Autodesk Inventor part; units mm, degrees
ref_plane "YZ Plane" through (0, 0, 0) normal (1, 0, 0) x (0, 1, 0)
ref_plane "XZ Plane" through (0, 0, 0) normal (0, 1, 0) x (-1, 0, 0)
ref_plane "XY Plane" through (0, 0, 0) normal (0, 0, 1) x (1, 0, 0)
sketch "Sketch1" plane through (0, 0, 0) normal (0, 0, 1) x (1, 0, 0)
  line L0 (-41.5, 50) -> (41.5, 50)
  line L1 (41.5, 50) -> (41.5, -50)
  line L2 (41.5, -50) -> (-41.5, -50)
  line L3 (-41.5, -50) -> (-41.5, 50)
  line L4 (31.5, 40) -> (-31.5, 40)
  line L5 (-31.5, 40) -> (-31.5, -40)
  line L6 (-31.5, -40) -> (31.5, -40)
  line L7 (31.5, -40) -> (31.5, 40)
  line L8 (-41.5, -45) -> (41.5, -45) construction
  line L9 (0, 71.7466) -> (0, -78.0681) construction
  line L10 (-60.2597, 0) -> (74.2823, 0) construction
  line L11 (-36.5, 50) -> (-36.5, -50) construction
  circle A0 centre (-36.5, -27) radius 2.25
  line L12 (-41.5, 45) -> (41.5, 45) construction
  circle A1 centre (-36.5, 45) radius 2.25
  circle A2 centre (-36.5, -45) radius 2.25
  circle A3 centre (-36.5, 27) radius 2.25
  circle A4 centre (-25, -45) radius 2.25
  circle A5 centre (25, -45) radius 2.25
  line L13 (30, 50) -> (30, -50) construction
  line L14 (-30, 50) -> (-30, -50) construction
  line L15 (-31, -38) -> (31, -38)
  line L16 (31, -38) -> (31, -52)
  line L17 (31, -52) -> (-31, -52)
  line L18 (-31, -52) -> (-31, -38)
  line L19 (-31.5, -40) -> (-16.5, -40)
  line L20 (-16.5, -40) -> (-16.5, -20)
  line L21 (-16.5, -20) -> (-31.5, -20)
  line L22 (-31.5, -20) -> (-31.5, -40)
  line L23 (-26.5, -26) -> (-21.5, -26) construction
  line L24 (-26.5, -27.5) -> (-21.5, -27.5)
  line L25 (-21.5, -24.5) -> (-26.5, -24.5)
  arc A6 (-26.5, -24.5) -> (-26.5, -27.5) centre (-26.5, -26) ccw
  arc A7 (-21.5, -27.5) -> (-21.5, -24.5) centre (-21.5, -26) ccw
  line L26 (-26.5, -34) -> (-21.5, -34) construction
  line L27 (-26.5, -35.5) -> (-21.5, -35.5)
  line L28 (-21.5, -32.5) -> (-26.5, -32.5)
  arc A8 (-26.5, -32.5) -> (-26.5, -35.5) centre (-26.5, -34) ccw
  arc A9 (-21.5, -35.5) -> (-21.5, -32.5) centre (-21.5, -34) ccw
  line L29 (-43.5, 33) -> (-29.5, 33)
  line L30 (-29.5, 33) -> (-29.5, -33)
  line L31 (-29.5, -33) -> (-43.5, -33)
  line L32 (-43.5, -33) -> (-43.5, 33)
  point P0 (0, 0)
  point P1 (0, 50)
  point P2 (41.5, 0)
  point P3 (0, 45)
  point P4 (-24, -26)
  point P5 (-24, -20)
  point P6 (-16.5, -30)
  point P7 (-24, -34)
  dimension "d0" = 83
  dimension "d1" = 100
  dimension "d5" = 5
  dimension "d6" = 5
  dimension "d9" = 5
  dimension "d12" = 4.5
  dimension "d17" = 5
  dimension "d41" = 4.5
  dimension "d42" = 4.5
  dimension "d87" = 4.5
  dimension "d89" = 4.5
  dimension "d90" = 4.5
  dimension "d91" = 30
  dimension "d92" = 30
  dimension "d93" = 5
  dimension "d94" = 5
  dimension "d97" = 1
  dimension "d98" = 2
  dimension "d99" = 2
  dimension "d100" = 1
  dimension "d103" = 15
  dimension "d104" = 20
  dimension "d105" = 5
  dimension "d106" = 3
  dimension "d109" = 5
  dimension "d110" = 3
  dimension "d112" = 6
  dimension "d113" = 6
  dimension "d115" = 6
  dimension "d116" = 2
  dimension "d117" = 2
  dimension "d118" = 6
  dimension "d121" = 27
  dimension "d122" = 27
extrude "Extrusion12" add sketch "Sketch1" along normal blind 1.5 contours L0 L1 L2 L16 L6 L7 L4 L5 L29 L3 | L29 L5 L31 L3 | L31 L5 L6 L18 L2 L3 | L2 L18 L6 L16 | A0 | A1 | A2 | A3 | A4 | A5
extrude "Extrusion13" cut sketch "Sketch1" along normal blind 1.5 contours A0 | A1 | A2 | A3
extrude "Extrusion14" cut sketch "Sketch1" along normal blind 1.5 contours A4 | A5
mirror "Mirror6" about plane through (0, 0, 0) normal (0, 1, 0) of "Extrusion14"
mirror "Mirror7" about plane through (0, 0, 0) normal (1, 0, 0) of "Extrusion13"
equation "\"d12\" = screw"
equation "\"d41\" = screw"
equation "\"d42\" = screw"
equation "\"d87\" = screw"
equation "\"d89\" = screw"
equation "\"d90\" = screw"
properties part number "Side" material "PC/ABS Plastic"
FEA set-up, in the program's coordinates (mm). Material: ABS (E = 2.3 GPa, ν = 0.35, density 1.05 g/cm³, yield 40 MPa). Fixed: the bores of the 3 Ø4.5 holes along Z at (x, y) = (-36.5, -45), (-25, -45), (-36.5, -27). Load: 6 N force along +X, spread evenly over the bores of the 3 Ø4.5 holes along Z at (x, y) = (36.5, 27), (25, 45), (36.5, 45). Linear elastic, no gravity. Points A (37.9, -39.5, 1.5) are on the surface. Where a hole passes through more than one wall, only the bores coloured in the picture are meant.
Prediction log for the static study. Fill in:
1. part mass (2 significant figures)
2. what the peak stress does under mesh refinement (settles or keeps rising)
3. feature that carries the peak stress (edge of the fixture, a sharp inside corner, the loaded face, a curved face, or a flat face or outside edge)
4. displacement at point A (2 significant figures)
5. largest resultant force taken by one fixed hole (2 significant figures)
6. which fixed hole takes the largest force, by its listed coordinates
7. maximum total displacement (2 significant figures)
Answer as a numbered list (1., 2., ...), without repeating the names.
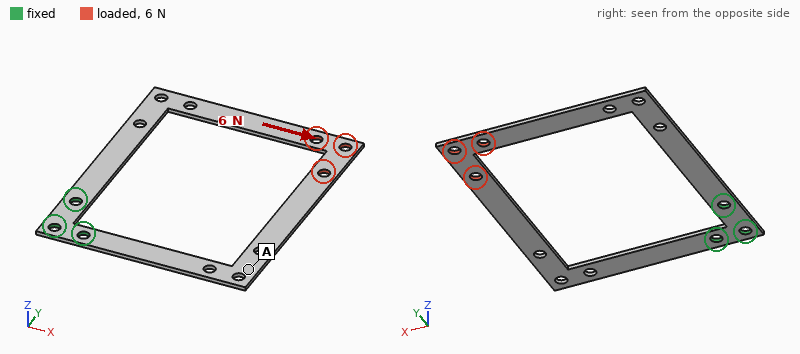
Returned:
1. 4.8 g
2. keeps rising
3. edge of the fixture
4. 0.71 mm
5. 9.2 N
6. (-36.5, -27)
7. 1.5 mm
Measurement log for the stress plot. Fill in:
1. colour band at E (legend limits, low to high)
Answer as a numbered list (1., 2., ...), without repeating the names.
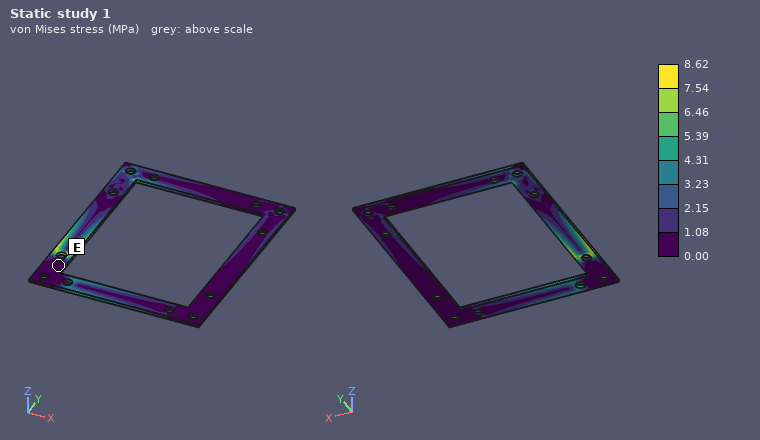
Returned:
1. 0.00 to 1.08 MPa
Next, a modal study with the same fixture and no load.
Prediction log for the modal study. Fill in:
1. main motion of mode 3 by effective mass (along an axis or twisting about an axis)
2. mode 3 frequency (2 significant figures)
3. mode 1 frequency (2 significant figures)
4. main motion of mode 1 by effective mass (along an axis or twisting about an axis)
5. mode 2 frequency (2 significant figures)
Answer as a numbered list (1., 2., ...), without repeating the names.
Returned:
1. along Z
2. 100 Hz
3. 25 Hz
4. along Z
5. 55 Hz
